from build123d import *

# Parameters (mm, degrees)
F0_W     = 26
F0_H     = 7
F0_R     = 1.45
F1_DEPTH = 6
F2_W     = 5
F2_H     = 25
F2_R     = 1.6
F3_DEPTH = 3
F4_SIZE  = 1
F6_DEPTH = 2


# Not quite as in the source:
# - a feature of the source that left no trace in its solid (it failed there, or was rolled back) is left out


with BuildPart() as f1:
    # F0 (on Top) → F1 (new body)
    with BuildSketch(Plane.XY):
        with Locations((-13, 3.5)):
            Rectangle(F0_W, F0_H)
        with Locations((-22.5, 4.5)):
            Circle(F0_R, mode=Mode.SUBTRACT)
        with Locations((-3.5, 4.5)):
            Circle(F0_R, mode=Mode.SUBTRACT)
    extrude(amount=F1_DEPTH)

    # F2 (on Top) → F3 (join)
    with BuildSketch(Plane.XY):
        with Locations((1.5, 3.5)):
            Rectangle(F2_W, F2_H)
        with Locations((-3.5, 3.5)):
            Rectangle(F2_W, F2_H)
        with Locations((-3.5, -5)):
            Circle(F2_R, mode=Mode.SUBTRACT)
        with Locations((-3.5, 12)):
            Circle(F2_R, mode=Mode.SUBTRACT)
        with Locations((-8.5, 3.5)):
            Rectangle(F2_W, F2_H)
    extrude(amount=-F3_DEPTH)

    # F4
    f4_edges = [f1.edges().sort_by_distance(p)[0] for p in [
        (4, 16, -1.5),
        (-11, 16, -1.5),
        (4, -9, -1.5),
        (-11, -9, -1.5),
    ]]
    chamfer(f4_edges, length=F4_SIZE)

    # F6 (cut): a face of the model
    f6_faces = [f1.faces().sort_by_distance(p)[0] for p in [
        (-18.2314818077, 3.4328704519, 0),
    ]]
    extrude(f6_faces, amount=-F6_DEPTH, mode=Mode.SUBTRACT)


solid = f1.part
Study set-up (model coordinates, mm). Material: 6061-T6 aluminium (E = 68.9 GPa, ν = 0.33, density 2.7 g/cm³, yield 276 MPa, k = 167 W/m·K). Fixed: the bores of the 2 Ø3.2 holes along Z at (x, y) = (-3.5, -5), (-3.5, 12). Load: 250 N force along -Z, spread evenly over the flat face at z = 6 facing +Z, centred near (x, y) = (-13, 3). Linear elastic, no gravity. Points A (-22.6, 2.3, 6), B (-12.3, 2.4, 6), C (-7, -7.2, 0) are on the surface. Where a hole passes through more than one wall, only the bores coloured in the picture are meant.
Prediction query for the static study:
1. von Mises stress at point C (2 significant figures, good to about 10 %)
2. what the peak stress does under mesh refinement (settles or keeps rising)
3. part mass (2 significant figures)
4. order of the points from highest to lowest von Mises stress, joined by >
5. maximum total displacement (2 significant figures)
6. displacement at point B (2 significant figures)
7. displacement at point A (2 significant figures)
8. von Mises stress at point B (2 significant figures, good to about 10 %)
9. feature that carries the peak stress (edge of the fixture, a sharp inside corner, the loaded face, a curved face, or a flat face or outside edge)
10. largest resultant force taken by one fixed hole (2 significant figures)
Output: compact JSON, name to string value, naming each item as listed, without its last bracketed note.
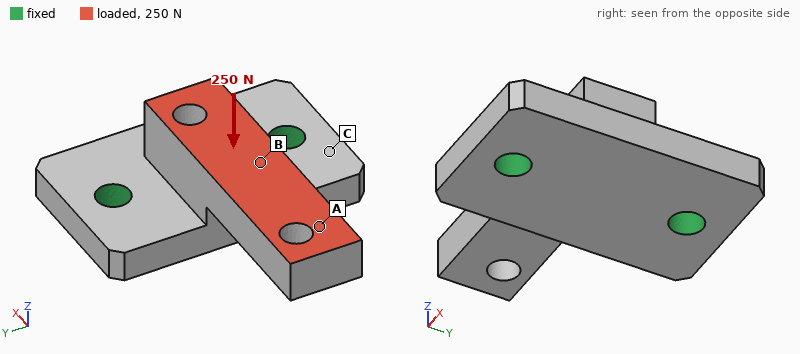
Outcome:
{"von Mises stress at point C": "24 MPa", "what the peak stress does under mesh refinement": "keeps rising", "part mass": "5.1 g", "order of the points from highest to lowest von Mises stress, joined by >": "B > C > A", "maximum total displacement": "86 µm", "displacement at point B": "28 µm", "displacement at point A": "70 µm", "von Mises stress at point B": "45 MPa", "feature that carries the peak stress": "edge of the fixture", "largest resultant force taken by one fixed hole": "140 N"}
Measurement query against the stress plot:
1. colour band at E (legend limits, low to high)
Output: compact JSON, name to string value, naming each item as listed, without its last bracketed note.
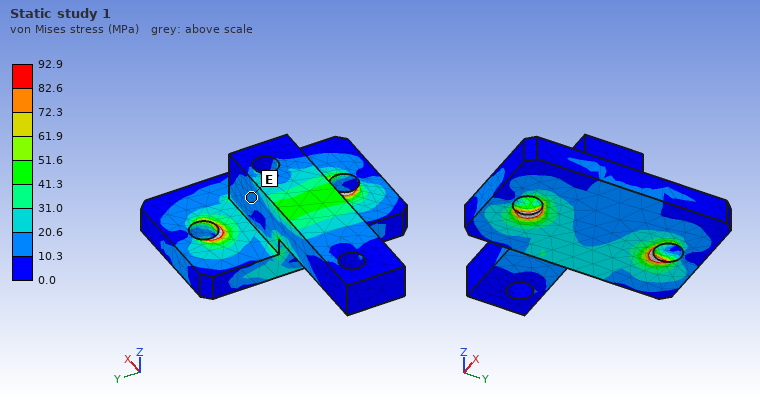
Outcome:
{"colour band at E": "10.3 to 20.6 MPa"}
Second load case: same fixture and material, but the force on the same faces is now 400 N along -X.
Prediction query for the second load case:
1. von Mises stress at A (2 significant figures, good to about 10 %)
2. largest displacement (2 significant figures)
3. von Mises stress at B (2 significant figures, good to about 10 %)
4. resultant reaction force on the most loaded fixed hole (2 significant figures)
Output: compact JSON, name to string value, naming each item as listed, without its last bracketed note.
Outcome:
{"von Mises stress at A": "11 MPa", "largest displacement": "81 µm", "von Mises stress at B": "30 MPa", "resultant reaction force on the most loaded fixed hole": "200 N"}
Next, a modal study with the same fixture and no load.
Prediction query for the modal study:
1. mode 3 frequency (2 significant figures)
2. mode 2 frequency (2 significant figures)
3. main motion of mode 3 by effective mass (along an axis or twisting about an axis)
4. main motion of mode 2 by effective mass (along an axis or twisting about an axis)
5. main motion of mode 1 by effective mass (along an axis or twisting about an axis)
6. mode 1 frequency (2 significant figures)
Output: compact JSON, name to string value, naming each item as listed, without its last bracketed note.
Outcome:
{"mode 3 frequency": "22 kHz", "mode 2 frequency": "13 kHz", "main motion of mode 3 by effective mass": "along X", "main motion of mode 2 by effective mass": "along Y", "main motion of mode 1 by effective mass": "along Z", "mode 1 frequency": "7700 Hz"}
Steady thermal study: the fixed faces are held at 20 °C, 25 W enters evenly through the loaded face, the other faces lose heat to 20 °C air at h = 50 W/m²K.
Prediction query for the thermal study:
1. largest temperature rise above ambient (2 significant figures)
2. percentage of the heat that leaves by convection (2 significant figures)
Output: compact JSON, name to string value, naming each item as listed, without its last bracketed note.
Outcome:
{"largest temperature rise above ambient": "52 K", "percentage of the heat that leaves by convection": "4.3 %"}
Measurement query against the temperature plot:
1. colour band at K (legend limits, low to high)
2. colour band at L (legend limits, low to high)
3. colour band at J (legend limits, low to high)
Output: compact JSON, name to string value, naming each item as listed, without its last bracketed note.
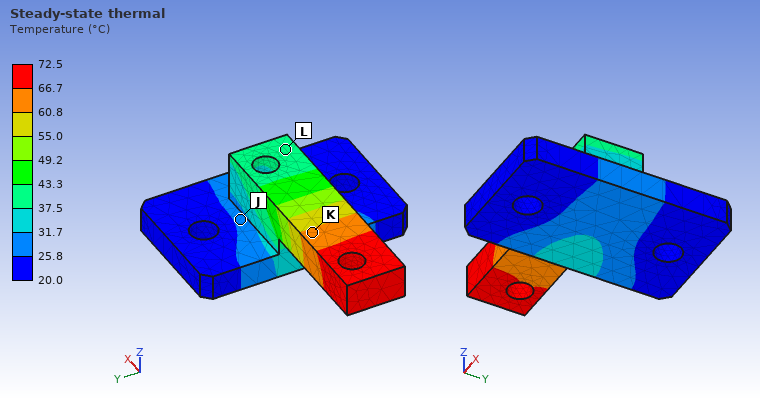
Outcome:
{"colour band at K": "60.8 to 66.7 °C", "colour band at L": "37.5 to 43.3 °C", "colour band at J": "25.8 to 31.7 °C"}
